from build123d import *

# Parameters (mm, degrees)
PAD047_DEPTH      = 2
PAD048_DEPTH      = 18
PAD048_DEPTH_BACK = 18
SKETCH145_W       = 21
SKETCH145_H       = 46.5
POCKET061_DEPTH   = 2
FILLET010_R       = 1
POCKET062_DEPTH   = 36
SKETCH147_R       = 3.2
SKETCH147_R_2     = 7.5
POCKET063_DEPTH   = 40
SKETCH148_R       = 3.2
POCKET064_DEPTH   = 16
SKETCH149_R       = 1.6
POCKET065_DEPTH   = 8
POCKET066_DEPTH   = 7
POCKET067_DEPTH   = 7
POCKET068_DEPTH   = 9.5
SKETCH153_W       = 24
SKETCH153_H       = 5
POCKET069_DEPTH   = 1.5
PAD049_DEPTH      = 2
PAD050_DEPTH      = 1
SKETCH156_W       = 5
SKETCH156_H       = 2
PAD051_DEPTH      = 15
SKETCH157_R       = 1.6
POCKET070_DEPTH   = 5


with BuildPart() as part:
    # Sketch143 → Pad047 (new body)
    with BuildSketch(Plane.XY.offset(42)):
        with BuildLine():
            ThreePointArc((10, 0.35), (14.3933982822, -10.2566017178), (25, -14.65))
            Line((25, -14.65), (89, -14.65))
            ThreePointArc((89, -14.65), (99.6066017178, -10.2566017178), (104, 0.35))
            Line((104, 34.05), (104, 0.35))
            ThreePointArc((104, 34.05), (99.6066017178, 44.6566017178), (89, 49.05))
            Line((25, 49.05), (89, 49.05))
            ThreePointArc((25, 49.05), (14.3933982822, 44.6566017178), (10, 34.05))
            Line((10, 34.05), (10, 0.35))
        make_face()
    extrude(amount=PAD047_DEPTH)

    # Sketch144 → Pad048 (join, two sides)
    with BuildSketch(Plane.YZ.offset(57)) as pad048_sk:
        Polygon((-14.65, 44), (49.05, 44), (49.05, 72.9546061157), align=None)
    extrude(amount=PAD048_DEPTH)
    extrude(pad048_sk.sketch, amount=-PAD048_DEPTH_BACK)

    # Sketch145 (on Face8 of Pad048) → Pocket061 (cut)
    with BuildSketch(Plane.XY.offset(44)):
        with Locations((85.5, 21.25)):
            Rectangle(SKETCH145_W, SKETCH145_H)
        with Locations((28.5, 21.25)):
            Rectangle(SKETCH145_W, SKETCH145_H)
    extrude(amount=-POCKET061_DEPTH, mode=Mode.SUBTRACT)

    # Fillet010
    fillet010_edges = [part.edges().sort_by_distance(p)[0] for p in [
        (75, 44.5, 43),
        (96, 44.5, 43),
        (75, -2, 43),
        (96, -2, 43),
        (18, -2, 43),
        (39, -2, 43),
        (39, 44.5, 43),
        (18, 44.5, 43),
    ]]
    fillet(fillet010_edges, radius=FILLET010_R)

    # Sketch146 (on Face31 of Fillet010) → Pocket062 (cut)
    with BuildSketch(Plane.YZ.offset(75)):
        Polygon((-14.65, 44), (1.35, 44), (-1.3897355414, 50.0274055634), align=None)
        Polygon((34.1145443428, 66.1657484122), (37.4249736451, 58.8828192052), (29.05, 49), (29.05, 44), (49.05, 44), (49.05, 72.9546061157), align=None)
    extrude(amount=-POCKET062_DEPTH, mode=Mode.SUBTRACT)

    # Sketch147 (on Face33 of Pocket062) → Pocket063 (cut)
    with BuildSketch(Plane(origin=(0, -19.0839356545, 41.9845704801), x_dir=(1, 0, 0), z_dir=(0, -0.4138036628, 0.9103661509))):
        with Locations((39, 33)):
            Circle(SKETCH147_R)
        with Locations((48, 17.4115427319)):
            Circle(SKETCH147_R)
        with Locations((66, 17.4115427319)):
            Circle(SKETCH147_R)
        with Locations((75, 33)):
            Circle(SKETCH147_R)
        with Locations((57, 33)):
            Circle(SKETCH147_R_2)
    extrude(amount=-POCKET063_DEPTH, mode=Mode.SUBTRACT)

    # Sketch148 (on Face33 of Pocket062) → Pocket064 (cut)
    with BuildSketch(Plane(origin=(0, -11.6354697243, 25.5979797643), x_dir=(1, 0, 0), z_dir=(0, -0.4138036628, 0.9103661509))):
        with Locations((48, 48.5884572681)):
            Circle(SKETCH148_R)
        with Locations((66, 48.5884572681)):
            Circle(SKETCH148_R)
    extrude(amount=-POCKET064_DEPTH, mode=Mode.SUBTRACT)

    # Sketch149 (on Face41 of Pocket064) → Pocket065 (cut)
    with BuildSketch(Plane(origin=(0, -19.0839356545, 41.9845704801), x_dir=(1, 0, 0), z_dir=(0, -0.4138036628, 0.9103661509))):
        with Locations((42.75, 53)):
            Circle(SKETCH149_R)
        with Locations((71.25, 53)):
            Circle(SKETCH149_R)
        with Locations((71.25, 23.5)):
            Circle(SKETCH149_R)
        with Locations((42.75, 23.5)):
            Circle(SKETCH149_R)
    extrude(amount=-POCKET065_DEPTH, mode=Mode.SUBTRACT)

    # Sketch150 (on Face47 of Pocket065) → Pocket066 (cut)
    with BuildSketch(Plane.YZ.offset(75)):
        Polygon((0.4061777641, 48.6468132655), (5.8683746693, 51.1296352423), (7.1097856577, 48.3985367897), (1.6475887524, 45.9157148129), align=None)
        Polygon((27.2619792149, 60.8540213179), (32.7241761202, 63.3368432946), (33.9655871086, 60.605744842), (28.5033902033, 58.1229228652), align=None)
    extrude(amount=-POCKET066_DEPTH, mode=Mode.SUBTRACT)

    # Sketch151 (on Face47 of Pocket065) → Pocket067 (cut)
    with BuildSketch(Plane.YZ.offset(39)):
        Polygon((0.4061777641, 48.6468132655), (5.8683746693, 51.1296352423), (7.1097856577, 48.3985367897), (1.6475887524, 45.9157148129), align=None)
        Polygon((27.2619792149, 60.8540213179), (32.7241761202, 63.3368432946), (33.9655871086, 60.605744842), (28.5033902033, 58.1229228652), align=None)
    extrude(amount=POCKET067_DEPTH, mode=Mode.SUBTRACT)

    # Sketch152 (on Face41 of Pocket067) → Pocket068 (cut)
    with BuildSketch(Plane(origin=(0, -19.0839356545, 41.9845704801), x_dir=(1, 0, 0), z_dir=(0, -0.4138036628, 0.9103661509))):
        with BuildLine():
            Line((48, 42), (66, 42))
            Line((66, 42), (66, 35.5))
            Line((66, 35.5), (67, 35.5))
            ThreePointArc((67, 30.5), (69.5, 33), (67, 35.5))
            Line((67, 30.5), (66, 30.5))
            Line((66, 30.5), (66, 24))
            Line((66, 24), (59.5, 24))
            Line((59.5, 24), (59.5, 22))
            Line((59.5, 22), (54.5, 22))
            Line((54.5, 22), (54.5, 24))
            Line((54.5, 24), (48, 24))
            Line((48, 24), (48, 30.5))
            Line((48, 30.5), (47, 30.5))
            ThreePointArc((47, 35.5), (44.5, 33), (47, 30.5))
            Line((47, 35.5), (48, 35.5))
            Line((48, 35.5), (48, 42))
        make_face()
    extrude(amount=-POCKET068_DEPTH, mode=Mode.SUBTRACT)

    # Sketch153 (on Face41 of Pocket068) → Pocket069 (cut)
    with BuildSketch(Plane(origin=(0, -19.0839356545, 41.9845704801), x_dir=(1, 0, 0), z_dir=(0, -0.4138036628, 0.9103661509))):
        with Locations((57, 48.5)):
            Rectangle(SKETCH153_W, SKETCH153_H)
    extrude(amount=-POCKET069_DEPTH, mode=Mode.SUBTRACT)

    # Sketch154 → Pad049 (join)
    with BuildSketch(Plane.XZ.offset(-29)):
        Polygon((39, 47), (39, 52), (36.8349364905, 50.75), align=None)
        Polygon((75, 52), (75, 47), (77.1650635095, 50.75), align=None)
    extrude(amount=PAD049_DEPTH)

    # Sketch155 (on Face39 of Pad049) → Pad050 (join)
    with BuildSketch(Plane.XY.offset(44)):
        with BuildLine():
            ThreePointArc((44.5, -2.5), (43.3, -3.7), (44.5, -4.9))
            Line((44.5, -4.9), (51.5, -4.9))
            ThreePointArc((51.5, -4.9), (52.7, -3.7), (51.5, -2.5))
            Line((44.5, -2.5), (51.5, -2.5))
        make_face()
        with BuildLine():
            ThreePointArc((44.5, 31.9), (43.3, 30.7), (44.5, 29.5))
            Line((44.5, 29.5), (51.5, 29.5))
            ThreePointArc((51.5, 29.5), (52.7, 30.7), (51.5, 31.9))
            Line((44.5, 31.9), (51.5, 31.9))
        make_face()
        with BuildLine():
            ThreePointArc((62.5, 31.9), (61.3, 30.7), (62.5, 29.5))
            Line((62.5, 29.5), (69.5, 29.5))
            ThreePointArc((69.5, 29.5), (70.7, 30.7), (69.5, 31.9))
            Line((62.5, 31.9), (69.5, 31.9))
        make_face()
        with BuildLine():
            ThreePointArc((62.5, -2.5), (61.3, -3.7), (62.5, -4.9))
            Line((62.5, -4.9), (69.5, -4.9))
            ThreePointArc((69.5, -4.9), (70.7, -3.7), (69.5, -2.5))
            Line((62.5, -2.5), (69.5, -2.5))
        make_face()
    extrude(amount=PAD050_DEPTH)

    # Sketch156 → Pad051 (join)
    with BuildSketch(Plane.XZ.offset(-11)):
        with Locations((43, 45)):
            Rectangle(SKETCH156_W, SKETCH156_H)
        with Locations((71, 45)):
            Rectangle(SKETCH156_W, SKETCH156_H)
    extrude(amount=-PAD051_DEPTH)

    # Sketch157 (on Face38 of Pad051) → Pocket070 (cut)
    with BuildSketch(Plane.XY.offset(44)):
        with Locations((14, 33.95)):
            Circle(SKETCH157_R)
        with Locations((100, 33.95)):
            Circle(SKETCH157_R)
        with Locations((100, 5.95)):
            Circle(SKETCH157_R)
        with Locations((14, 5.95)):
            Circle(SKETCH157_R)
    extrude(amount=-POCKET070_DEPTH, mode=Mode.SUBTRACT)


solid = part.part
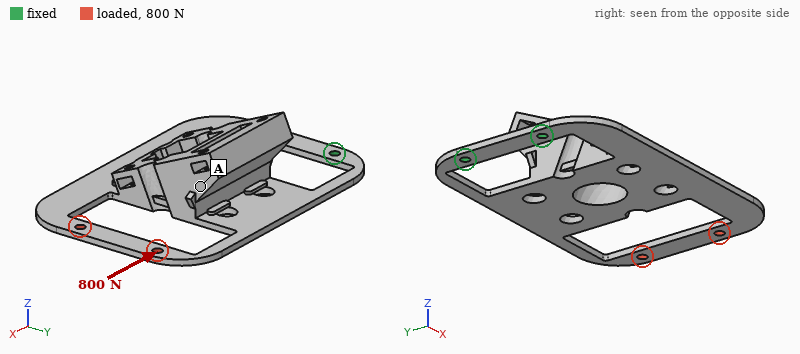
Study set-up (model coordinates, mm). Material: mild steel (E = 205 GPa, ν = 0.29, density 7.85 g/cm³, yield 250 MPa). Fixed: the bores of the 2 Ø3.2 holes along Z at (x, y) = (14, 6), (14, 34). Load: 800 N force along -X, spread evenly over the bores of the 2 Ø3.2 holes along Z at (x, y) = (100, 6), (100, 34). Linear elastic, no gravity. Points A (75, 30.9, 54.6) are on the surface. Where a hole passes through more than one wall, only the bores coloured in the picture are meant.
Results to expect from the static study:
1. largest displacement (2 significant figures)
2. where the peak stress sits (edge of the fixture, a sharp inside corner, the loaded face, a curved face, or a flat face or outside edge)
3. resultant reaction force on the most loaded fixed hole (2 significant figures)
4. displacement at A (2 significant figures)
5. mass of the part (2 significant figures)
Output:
80 µm
a curved face
420 N
24 µm
150 g
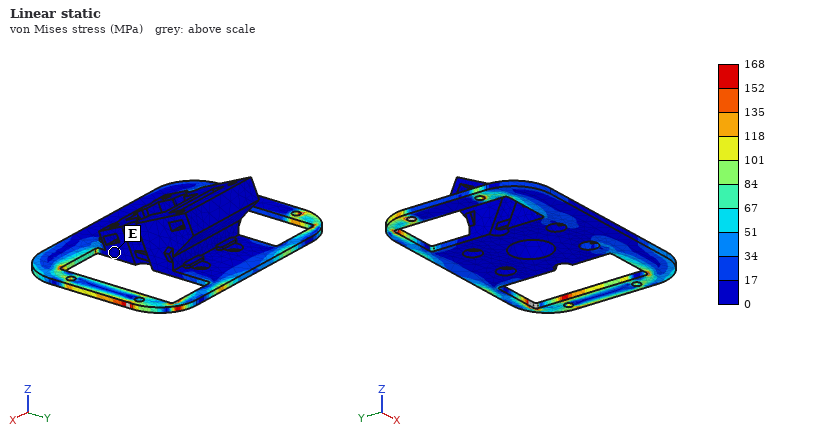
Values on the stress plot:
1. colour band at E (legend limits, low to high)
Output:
0 to 17 MPa
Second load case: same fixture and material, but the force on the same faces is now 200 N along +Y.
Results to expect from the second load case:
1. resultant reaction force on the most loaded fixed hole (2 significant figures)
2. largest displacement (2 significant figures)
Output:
430 N
0.16 mm
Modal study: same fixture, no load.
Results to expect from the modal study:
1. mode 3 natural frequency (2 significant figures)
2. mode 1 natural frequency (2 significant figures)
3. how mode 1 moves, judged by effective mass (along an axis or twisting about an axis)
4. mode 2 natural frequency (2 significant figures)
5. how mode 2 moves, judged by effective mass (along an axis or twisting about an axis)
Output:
660 Hz
84 Hz
along Z
390 Hz
along Y
